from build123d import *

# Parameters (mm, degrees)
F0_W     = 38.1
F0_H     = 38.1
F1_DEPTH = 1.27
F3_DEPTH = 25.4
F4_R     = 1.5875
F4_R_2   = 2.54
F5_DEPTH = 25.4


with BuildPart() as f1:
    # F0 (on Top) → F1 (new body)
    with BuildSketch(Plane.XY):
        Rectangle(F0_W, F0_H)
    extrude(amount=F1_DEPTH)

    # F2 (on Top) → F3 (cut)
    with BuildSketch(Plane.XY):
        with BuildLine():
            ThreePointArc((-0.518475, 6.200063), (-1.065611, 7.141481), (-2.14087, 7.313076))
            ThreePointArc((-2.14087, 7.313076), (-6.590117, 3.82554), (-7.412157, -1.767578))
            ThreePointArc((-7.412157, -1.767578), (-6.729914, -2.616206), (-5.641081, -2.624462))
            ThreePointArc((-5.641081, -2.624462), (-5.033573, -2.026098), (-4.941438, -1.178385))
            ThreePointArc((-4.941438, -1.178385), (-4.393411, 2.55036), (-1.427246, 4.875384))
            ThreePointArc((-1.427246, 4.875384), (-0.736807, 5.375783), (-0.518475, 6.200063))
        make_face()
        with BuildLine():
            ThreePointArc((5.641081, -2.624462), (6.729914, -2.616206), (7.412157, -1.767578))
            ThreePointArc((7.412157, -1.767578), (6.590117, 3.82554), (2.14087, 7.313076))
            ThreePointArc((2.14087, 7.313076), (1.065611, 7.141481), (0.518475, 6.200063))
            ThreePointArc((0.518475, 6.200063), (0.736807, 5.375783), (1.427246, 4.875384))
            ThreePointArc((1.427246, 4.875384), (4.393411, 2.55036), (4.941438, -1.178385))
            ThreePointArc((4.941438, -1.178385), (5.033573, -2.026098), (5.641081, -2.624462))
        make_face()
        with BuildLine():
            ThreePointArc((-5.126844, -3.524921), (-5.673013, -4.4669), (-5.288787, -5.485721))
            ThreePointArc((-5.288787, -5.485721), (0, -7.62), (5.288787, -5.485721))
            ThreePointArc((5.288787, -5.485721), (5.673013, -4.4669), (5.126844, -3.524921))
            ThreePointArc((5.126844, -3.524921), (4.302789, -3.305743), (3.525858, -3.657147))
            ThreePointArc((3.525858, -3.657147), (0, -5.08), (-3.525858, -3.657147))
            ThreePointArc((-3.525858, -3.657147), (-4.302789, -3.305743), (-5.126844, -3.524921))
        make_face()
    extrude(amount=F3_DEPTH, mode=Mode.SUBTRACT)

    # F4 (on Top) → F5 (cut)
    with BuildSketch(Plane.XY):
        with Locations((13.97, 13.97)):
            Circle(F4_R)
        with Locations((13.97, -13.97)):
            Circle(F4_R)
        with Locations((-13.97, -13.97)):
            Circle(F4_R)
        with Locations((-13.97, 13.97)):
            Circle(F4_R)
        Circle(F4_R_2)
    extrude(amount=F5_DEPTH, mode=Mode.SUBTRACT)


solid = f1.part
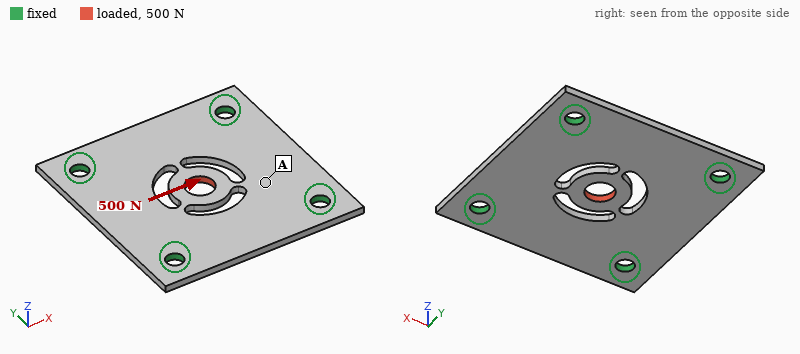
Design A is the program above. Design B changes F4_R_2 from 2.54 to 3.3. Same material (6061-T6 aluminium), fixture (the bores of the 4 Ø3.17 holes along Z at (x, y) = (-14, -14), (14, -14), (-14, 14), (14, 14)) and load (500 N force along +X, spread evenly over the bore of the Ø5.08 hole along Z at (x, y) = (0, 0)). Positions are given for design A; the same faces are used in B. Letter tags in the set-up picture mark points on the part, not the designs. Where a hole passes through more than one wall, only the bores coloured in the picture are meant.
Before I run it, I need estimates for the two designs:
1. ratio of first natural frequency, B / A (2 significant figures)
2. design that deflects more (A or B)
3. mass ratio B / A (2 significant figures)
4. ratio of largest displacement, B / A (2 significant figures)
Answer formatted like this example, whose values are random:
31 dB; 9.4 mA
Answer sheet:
1.0; B; 0.99; 1.7
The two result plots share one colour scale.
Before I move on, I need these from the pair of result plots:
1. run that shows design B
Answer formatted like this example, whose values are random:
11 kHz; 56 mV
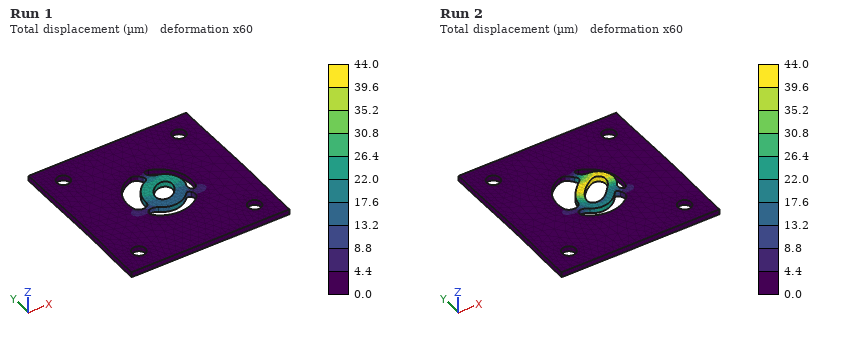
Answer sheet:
Run 2
